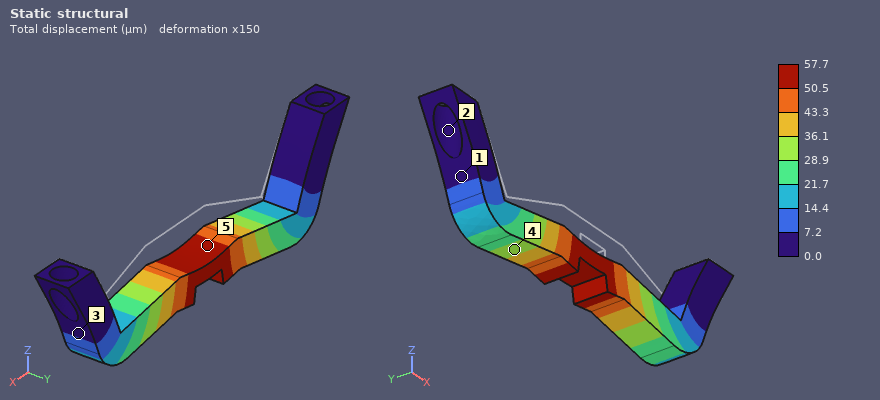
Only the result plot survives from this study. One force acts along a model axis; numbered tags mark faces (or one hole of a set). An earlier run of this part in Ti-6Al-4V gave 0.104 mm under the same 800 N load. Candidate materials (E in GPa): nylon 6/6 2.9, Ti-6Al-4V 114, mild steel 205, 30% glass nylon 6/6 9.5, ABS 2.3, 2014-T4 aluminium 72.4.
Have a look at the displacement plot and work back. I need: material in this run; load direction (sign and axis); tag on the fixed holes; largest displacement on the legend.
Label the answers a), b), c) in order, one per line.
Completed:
a) mild steel
b) -Z
c) 2
d) 57.7 µm
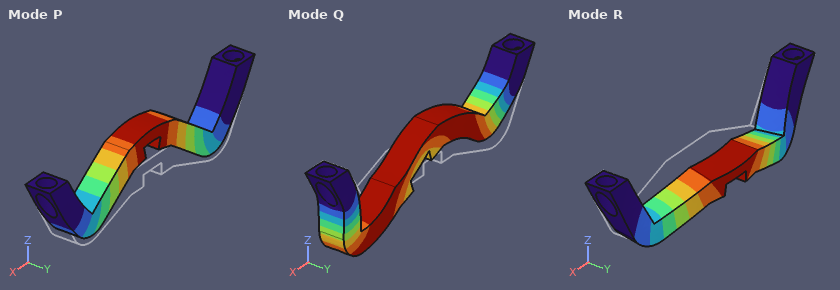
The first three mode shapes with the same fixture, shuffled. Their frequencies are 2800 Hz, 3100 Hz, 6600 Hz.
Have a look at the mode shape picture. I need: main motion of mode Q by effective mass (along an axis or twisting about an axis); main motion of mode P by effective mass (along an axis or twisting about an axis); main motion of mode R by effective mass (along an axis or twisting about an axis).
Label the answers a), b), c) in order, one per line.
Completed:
a) along X
b) along Z
c) along Y
